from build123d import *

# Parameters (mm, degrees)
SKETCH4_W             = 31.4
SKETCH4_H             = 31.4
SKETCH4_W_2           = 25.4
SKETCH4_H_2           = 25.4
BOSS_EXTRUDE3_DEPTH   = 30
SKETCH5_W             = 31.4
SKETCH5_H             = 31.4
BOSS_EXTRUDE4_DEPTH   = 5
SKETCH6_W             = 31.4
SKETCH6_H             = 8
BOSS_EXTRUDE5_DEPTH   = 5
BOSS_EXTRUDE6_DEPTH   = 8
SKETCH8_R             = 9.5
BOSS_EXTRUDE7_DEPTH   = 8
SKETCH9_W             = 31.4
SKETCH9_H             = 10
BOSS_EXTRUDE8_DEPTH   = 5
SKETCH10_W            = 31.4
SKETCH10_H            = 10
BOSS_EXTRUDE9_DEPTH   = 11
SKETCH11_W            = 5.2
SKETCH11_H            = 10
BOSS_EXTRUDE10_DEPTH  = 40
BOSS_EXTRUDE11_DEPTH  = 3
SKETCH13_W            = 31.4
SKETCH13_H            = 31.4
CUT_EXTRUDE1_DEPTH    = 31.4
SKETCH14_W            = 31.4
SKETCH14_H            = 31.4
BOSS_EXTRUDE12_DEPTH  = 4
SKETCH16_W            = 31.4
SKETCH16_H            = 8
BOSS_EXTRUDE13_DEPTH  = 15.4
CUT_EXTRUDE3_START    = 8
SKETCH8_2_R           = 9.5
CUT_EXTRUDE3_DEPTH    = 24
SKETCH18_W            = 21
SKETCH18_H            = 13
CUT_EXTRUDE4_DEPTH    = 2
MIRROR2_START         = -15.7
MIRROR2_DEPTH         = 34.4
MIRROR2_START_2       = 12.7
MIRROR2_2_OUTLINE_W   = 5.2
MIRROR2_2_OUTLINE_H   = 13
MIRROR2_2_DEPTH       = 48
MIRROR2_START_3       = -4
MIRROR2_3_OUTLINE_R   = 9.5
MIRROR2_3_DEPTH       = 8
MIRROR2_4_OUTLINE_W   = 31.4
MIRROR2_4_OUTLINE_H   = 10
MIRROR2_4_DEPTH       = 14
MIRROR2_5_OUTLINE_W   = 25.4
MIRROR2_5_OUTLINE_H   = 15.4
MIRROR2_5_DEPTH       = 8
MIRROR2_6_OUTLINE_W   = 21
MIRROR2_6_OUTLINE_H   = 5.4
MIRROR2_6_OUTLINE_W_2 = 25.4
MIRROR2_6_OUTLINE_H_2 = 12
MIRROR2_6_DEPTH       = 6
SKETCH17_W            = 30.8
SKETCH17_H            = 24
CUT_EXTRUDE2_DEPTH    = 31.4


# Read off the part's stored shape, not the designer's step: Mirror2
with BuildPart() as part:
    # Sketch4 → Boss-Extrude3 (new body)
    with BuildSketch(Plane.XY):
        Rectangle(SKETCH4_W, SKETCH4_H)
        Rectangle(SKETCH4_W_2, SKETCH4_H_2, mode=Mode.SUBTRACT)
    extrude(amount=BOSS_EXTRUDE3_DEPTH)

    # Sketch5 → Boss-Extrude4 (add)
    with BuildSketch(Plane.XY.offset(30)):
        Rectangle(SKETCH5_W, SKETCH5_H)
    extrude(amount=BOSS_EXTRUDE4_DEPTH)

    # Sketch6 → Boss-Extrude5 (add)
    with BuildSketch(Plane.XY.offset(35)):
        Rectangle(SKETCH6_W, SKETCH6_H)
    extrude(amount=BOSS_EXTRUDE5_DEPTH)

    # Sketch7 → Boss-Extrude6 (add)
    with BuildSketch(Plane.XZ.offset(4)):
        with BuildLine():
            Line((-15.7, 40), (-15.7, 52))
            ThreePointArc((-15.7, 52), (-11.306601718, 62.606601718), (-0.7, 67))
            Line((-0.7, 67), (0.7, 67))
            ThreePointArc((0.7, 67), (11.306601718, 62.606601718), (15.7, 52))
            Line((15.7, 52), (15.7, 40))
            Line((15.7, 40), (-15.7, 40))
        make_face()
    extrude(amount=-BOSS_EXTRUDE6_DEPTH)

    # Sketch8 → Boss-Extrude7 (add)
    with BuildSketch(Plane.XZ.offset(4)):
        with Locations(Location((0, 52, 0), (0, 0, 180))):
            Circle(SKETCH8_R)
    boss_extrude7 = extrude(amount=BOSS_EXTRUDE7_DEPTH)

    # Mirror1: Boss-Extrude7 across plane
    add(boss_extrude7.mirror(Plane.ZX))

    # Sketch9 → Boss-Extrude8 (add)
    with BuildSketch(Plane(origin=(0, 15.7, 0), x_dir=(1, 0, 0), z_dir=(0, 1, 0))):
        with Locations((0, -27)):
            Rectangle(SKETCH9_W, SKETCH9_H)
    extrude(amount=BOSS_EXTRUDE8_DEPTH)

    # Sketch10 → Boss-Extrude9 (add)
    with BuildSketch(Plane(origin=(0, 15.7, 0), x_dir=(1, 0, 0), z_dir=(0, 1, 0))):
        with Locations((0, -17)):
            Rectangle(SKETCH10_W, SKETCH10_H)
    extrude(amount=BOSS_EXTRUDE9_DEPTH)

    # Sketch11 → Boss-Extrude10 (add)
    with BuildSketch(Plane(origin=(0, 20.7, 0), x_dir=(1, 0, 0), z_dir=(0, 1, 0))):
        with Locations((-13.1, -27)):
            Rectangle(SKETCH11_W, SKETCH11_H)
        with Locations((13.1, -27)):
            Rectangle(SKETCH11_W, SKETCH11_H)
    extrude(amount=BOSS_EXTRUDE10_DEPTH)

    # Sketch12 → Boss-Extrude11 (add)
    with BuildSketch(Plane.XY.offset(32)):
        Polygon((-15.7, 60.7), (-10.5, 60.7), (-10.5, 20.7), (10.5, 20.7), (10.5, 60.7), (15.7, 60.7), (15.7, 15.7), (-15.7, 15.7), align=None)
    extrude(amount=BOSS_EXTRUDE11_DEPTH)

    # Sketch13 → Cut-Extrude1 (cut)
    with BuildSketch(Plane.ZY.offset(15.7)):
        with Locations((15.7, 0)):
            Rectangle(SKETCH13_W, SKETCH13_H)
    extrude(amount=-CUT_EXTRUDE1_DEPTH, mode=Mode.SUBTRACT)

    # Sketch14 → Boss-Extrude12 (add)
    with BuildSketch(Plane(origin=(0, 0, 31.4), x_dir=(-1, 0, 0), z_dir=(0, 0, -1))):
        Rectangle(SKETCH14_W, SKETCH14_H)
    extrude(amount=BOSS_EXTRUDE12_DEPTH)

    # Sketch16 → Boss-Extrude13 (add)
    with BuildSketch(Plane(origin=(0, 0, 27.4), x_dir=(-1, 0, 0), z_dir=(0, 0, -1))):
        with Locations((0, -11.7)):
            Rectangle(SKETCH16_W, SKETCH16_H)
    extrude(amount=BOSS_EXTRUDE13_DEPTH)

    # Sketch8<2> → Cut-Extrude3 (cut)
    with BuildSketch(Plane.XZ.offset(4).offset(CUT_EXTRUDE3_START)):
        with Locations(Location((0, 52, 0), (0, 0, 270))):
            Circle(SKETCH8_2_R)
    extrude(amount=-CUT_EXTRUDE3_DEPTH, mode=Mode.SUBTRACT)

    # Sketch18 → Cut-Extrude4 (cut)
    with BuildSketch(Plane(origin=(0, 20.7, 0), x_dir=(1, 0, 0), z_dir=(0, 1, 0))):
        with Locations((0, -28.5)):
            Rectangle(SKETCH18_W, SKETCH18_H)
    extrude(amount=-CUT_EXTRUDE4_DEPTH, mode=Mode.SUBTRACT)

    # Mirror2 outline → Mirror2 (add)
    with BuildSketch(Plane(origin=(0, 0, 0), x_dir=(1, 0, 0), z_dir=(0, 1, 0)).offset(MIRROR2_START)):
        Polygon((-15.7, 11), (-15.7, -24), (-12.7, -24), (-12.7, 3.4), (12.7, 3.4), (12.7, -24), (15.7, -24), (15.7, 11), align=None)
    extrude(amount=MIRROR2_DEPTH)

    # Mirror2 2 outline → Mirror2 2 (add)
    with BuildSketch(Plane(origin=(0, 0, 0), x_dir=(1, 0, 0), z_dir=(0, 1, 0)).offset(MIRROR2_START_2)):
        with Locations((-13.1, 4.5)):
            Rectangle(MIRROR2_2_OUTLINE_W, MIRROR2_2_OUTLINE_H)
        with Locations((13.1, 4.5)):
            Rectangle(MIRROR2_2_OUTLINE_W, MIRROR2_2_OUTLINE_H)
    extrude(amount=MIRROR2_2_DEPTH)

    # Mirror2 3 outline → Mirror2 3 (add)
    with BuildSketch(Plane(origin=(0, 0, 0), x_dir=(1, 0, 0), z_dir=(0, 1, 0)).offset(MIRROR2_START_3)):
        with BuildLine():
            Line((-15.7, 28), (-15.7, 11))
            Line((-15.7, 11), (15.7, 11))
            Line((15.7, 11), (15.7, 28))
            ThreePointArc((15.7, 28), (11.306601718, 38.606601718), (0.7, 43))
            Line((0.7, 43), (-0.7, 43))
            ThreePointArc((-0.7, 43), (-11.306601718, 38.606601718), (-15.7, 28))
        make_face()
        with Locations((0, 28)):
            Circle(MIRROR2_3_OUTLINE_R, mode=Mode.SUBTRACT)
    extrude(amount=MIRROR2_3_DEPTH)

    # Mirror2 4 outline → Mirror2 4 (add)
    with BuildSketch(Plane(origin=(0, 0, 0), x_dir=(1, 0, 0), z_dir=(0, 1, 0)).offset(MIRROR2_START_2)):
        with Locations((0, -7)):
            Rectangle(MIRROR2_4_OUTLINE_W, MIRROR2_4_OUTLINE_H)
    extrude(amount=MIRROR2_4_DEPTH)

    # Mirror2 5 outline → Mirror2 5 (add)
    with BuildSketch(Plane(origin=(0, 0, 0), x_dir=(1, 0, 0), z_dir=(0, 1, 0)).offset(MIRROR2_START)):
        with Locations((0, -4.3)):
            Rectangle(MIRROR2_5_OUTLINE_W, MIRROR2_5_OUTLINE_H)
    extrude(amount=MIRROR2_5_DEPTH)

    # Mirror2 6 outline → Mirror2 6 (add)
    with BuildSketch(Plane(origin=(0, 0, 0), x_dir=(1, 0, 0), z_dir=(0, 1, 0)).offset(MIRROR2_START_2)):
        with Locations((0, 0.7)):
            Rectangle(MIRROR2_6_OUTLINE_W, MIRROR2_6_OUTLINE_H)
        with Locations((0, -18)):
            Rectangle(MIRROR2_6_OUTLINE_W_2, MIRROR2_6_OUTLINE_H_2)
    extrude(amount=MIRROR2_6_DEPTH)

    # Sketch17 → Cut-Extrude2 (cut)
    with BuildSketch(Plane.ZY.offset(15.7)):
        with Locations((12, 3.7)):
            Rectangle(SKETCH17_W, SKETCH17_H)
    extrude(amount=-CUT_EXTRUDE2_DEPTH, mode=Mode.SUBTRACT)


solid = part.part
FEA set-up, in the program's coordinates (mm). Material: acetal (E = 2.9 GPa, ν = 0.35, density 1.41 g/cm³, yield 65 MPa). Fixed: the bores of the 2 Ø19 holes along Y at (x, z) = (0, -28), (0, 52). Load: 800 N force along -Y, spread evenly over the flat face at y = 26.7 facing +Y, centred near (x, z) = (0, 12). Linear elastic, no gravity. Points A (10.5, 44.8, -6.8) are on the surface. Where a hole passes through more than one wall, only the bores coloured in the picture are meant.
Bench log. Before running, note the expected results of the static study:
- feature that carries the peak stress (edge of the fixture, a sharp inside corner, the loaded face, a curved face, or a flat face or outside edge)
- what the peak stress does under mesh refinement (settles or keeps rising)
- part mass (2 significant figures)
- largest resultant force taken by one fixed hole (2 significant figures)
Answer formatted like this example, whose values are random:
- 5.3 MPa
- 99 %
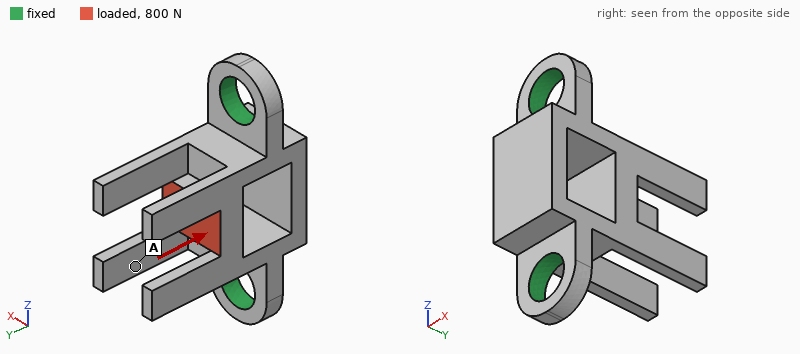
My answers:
- edge of the fixture
- keeps rising
- 75 g
- 420 N
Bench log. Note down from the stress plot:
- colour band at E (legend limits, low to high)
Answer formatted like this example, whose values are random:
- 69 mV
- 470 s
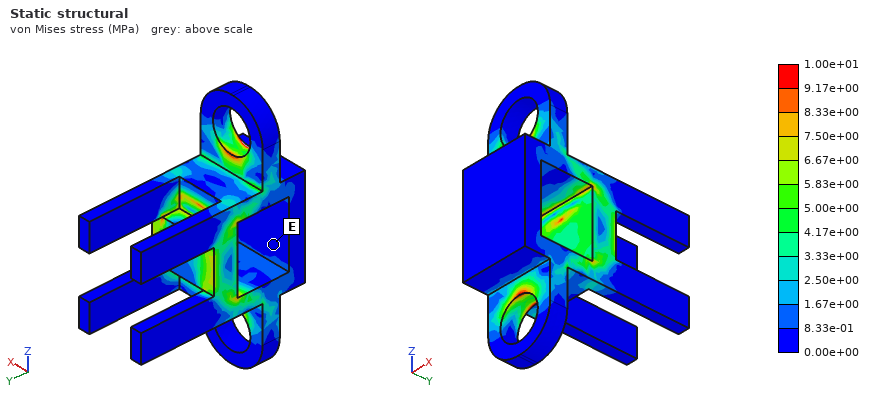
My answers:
- 0.00e+00 to 8.33e-01 MPa
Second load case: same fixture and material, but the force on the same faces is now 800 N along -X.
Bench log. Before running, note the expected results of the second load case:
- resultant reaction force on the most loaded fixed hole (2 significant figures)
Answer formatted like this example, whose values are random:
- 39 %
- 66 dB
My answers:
- 400 N
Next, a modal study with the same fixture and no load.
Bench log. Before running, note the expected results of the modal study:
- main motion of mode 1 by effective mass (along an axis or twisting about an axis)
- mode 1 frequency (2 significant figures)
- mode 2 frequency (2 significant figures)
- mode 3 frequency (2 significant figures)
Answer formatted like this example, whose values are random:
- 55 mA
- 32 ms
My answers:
- along X
- 590 Hz
- 700 Hz
- 720 Hz
